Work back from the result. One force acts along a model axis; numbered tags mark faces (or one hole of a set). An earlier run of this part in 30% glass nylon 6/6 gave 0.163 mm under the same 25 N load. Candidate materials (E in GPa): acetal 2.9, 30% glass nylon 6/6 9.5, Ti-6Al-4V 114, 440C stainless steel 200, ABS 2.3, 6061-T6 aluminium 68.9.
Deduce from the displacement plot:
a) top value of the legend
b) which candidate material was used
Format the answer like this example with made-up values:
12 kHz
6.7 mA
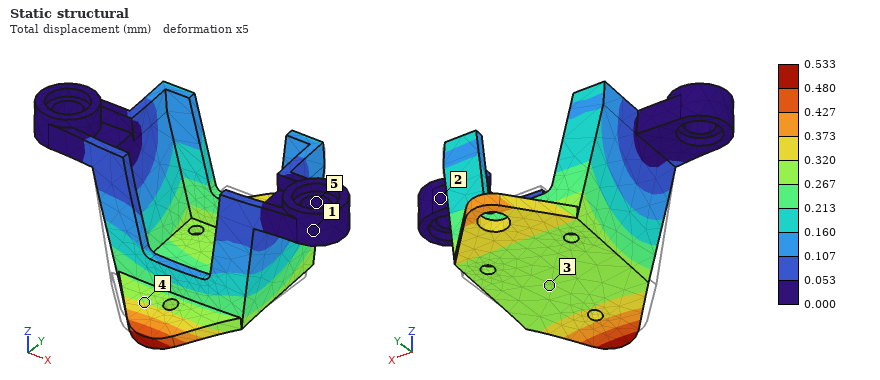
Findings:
0.533 mm
acetal
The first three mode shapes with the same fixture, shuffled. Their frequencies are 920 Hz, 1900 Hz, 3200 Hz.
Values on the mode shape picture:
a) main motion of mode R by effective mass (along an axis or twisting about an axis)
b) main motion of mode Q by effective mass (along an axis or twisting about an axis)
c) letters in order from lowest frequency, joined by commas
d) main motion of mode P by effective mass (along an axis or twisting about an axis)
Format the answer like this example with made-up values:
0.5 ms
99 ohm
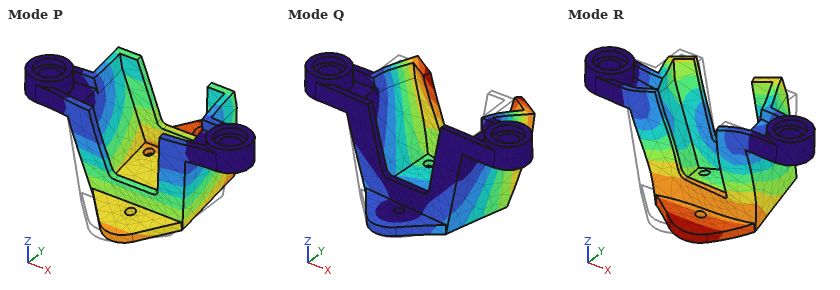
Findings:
along X
along X
P, Q, R
along Y
